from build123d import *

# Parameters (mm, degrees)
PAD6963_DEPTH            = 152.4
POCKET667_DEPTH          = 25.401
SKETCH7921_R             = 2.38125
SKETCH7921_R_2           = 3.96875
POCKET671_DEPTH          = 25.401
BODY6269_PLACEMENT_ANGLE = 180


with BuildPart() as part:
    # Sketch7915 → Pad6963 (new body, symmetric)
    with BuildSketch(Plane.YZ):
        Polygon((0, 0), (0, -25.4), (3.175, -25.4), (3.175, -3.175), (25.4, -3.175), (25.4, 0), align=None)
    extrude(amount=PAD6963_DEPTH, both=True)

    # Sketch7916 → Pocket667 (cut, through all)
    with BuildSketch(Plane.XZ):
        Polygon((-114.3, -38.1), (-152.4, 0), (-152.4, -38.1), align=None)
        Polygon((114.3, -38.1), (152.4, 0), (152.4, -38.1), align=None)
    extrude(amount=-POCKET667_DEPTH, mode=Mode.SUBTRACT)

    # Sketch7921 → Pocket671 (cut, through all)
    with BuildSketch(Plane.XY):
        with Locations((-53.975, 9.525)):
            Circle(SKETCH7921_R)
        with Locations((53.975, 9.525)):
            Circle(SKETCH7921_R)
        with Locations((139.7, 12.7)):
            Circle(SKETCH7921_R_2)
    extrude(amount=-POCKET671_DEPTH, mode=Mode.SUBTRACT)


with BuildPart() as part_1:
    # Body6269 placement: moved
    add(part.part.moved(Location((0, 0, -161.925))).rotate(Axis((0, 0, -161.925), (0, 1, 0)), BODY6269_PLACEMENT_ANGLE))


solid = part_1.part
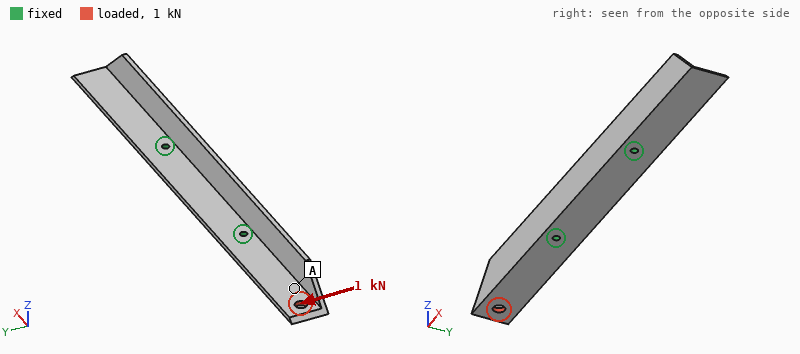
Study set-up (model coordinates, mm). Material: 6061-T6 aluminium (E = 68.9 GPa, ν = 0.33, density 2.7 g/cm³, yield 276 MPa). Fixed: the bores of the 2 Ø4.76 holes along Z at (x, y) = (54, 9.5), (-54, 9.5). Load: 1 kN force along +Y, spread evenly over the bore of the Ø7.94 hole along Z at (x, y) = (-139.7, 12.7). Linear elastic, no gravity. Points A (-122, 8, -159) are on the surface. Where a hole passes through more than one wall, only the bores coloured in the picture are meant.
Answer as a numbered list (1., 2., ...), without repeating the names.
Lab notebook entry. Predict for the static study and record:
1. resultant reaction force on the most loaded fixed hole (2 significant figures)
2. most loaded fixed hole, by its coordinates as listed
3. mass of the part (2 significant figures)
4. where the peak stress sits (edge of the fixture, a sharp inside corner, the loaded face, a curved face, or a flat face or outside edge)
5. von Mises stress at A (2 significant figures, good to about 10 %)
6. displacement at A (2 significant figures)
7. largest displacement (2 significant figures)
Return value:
1. 1.6 kN
2. (-54, 9.5)
3. 120 g
4. edge of the fixture
5. 28 MPa
6. 0.79 mm
7. 1.3 mm
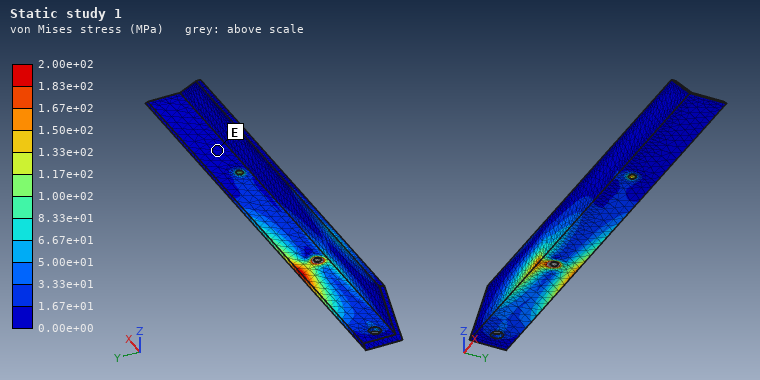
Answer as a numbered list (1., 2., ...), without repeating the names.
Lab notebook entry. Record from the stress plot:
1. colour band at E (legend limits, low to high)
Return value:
1. 0.00e+00 to 1.67e+01 MPa
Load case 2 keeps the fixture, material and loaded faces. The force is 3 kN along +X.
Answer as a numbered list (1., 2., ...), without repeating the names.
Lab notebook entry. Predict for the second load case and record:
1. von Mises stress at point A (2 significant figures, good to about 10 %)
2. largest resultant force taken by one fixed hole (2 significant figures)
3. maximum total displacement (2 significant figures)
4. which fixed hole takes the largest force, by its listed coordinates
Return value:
1. 29 MPa
2. 2.7 kN
3. 0.15 mm
4. (-54, 9.5)
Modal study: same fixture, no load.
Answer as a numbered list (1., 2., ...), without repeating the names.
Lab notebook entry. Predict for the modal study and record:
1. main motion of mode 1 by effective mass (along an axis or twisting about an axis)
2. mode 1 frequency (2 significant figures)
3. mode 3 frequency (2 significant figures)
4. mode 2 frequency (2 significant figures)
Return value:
1. along Z
2. 1100 Hz
3. 1100 Hz
4. 1100 Hz
